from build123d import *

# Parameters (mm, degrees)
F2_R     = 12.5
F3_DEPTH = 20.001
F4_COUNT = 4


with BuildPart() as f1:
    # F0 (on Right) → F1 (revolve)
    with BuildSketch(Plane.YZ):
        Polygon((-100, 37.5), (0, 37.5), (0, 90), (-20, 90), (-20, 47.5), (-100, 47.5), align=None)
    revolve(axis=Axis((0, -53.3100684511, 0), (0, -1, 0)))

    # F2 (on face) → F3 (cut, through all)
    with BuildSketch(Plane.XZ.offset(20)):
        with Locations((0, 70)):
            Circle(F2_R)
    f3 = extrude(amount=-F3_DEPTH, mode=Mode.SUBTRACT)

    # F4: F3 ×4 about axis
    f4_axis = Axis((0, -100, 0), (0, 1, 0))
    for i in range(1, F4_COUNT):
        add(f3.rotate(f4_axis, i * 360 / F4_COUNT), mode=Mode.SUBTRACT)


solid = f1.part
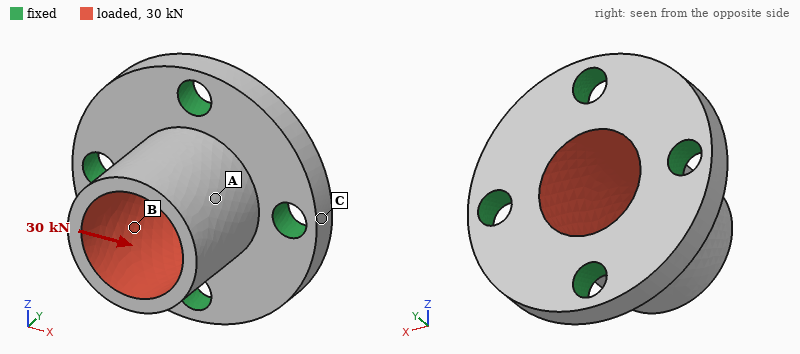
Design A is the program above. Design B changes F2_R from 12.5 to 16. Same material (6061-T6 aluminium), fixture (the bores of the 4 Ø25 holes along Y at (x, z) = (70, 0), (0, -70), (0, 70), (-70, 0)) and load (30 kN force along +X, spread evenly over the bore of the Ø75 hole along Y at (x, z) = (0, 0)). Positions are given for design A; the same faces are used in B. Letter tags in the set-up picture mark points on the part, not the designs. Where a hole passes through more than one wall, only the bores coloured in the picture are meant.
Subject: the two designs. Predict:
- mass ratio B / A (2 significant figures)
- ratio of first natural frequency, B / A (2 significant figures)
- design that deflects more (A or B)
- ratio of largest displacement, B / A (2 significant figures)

0.96
1.0
A
0.90
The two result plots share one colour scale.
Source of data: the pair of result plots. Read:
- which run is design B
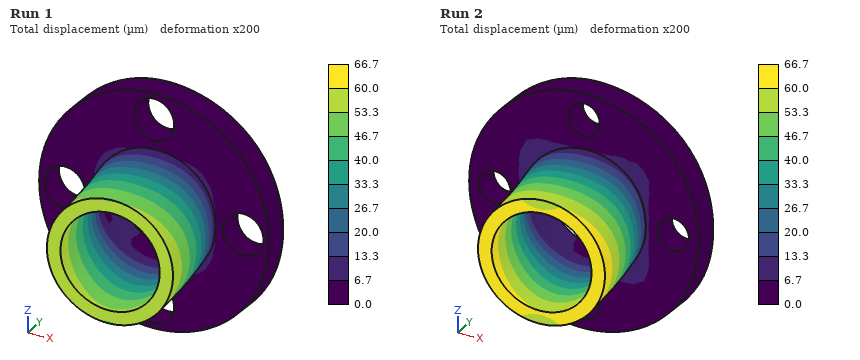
Run 1
